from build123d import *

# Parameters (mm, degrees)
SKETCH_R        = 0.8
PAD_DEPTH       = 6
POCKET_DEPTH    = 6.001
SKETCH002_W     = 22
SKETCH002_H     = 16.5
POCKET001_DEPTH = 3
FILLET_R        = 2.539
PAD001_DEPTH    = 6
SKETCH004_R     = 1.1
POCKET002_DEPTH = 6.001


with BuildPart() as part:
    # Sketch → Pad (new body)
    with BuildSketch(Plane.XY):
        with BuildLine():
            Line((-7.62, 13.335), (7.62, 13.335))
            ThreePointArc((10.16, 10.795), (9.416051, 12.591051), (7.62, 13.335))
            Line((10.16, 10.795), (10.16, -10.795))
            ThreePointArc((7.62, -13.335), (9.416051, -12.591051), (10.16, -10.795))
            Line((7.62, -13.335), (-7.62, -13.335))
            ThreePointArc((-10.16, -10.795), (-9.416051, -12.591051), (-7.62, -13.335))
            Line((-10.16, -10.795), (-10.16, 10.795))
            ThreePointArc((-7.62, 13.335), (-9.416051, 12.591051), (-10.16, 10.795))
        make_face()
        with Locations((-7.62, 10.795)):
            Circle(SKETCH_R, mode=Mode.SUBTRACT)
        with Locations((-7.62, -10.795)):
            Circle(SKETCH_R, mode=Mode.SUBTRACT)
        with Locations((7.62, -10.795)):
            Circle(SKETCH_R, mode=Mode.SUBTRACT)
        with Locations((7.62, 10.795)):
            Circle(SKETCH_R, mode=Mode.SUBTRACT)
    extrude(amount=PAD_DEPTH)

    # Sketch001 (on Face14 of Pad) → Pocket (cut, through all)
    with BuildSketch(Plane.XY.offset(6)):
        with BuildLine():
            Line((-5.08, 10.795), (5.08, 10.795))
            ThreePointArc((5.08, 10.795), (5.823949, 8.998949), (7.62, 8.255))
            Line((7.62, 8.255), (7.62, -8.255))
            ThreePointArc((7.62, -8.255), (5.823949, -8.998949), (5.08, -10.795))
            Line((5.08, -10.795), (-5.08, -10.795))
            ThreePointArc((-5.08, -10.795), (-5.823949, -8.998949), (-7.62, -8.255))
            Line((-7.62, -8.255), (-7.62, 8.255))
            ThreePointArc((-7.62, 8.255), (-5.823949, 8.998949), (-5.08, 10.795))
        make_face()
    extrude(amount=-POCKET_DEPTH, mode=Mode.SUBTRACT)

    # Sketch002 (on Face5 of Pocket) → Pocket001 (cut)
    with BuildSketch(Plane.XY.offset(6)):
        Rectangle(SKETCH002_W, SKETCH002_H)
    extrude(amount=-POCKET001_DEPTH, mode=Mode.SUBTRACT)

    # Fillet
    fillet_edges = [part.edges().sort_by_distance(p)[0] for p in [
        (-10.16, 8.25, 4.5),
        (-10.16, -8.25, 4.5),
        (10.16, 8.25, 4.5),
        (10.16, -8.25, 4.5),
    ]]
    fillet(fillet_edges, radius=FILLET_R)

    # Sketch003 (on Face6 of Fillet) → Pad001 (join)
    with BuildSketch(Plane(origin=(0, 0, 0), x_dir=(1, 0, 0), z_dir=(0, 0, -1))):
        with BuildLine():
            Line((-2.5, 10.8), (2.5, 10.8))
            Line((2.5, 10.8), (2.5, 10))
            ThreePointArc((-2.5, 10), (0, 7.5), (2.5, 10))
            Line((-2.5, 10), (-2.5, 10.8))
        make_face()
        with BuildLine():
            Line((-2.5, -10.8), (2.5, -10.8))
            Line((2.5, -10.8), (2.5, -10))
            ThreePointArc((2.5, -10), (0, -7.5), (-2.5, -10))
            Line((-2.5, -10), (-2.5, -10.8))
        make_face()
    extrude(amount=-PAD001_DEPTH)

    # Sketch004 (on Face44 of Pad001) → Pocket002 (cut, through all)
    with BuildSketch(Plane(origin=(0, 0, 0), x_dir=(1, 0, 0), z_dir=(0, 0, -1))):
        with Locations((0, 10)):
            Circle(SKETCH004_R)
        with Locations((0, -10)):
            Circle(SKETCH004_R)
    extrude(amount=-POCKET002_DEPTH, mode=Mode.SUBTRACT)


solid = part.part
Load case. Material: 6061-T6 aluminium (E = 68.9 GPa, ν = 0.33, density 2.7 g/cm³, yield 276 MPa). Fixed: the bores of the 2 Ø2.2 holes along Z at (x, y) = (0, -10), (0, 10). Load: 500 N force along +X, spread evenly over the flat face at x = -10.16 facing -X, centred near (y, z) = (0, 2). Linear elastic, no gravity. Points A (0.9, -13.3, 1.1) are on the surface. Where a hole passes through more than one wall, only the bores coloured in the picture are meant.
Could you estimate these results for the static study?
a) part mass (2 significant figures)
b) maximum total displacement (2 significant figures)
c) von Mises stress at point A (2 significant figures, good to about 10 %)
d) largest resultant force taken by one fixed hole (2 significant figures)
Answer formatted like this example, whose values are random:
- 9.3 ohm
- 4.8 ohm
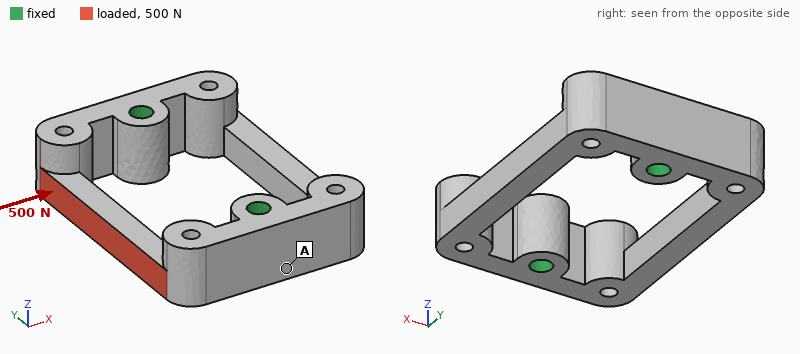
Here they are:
- 3.2 g
- 56 µm
- 24 MPa
- 320 N
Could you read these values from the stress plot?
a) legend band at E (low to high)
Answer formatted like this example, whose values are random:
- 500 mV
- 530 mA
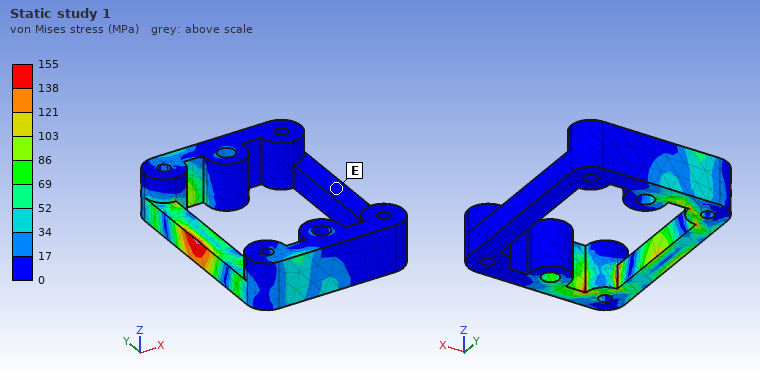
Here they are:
- 0 to 17 MPa
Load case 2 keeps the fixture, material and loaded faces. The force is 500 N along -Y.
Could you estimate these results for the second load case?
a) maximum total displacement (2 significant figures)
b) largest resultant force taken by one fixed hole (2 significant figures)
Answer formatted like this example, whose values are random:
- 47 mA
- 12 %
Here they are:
- 47 µm
- 270 N
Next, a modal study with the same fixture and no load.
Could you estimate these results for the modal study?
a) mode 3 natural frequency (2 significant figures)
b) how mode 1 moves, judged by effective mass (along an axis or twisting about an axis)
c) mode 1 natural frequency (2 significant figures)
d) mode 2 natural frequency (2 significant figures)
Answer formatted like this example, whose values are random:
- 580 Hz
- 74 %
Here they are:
- 18 kHz
- twisting about Y
- 17 kHz
- 18 kHz
